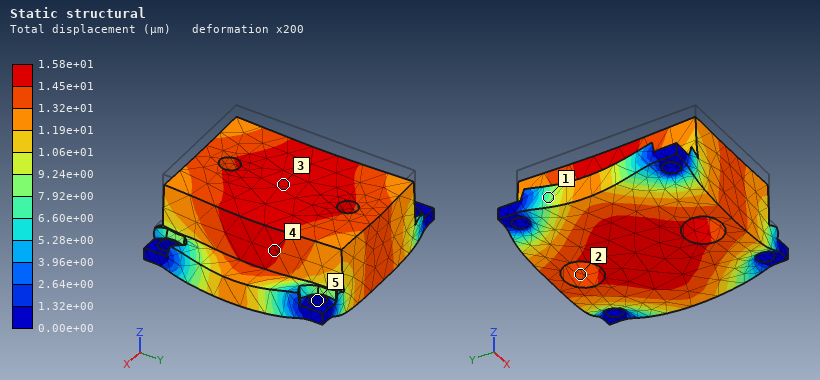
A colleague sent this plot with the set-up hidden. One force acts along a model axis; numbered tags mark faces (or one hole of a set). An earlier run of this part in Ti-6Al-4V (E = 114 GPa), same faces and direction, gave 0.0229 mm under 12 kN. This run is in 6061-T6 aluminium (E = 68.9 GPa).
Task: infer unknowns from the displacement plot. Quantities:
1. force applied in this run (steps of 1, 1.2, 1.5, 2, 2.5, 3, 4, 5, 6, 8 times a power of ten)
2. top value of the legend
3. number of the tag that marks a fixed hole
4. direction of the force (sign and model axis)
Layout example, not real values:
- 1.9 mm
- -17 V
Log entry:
- 5 kN
- 1.58e+01 µm
- 5
- -Z
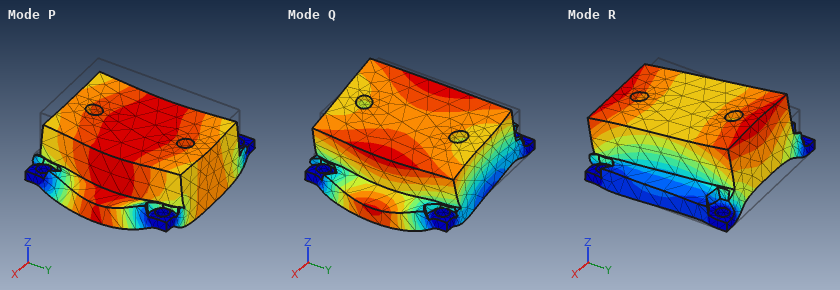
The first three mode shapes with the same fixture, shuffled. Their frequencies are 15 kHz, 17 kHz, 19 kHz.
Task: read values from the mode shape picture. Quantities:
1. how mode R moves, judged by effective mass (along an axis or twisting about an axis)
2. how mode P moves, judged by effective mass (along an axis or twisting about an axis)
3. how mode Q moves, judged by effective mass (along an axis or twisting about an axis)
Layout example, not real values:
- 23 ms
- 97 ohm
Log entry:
- along Y
- along Z
- along X
